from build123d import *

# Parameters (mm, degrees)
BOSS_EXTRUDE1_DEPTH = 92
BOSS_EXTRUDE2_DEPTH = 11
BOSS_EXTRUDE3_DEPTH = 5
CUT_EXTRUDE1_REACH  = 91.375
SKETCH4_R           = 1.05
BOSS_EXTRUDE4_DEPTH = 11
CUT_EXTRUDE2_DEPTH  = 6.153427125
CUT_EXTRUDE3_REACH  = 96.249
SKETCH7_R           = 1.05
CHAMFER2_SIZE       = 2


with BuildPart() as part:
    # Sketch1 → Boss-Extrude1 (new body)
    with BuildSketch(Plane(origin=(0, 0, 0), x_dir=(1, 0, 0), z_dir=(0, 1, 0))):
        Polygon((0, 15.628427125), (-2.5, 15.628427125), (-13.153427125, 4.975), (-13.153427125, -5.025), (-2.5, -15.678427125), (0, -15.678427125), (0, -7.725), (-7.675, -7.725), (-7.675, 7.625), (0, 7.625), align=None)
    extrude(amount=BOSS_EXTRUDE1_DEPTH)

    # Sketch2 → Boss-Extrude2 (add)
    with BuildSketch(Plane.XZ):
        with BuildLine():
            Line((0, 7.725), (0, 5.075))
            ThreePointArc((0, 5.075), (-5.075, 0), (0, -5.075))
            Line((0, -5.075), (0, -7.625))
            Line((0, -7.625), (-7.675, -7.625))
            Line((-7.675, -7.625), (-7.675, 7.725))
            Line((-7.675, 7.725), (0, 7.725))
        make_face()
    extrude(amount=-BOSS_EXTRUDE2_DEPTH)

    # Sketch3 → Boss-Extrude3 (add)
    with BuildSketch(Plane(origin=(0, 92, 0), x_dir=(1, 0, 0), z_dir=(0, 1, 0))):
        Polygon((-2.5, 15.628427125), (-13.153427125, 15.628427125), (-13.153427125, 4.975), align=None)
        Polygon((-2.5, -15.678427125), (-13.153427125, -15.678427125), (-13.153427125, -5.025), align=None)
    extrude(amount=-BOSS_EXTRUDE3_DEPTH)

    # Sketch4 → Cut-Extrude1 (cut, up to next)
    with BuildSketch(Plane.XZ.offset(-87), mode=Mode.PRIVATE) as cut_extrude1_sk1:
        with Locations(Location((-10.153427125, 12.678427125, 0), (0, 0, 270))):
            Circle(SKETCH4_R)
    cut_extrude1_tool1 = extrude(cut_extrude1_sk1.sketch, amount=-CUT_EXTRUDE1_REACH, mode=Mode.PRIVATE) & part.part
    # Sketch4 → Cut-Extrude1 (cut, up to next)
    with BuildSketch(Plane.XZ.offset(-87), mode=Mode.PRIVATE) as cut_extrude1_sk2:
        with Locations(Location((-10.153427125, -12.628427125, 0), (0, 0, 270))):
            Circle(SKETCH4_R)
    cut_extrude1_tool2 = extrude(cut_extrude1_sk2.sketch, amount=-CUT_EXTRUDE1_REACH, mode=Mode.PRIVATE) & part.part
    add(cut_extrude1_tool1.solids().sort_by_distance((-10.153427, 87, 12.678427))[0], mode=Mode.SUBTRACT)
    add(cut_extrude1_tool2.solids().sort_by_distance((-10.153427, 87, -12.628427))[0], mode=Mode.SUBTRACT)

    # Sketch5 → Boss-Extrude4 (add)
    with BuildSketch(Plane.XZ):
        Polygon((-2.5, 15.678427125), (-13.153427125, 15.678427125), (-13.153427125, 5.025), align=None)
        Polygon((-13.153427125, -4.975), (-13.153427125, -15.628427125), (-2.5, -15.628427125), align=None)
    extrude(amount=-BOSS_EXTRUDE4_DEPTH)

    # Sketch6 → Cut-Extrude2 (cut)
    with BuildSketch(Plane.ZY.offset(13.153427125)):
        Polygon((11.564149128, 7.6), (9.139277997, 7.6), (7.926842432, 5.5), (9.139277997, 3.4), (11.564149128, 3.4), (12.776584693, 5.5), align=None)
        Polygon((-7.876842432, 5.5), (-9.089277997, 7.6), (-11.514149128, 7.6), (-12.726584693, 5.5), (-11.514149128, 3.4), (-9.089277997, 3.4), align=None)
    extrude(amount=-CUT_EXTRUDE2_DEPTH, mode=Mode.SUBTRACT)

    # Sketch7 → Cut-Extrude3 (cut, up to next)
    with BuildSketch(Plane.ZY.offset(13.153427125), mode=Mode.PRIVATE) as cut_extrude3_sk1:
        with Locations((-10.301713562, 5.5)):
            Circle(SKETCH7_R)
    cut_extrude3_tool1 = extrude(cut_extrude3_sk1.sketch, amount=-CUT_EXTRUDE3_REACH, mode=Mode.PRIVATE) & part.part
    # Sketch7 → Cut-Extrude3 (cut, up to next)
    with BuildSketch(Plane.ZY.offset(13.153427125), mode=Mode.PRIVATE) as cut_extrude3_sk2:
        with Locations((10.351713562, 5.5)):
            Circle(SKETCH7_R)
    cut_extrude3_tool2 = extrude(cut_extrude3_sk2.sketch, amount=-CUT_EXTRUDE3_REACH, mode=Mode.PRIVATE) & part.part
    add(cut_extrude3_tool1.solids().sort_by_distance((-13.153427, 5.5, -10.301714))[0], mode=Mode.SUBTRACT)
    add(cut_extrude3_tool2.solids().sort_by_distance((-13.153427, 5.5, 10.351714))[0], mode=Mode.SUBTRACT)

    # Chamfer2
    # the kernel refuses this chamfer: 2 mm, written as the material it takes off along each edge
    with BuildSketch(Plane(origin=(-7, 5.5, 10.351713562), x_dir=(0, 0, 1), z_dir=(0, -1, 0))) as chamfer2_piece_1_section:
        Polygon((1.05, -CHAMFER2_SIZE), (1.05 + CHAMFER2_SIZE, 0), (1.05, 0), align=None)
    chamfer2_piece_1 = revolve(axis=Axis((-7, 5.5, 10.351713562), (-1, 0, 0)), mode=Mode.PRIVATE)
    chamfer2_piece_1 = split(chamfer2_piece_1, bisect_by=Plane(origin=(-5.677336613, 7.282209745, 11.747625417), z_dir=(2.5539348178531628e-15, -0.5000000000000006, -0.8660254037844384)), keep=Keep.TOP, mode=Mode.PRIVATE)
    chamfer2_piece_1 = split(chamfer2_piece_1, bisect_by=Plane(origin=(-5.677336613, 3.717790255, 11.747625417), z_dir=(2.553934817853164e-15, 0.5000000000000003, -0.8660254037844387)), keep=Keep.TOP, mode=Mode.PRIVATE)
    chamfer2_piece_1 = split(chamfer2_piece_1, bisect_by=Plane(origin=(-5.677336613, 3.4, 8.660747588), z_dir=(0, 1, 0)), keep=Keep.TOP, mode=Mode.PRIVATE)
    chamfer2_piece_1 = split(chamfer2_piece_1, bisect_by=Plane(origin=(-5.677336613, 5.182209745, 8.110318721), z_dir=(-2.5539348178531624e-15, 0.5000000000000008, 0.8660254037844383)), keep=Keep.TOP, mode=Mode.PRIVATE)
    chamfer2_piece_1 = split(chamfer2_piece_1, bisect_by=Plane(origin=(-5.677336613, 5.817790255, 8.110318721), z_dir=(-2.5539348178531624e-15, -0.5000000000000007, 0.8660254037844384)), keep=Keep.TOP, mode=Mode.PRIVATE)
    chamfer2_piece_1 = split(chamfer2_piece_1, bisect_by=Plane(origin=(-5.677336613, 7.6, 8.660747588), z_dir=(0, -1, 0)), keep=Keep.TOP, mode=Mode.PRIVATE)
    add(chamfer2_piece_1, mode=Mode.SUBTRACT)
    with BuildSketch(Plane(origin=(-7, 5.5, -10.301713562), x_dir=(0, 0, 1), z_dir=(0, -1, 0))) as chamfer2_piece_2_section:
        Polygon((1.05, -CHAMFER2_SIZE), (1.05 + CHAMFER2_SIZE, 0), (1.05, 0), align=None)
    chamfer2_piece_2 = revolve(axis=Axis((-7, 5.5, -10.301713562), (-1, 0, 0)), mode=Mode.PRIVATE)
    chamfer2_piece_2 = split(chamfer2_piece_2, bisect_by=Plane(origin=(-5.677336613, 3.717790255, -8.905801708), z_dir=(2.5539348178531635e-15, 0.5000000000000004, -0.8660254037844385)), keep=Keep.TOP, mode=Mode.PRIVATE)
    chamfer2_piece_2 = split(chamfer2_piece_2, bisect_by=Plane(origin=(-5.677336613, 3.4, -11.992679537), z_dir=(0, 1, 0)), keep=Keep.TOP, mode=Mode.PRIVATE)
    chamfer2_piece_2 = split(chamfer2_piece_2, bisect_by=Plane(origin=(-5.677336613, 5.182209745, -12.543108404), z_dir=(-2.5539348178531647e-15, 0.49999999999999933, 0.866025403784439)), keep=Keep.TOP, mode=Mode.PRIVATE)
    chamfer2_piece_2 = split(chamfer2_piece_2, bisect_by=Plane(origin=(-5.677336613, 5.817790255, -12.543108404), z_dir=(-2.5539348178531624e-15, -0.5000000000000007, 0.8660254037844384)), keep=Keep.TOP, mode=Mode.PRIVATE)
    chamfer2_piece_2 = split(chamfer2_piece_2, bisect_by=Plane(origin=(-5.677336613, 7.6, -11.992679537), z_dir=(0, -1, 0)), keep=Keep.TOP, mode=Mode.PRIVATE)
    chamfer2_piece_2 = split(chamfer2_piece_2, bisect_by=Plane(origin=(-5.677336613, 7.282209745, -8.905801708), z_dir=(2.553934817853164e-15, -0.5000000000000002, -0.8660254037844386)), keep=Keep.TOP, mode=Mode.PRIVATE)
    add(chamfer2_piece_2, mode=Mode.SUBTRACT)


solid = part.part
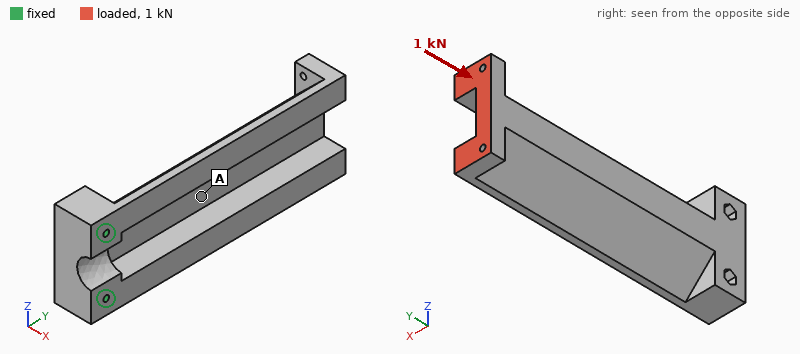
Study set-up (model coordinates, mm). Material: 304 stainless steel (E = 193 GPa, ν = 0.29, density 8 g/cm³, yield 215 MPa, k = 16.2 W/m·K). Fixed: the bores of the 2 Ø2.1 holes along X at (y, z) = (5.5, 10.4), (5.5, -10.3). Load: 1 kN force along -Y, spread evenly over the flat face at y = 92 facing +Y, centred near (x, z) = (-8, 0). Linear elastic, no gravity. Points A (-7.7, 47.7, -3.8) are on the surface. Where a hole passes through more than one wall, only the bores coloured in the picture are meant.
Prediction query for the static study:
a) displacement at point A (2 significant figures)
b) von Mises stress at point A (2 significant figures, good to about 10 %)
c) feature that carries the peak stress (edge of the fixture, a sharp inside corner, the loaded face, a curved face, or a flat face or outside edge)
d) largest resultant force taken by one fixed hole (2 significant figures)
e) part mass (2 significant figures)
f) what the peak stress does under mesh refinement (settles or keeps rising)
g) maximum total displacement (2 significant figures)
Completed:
14 µm
5.9 MPa
edge of the fixture
500 N
150 g
keeps rising
35 µm
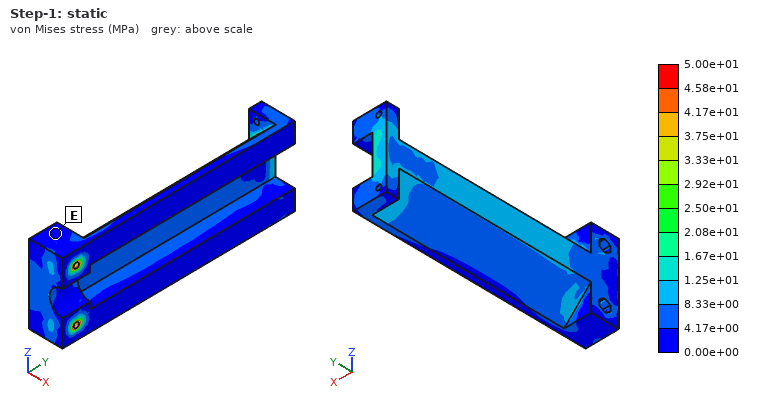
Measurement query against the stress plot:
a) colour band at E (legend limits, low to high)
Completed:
0.00e+00 to 4.17e+00 MPa
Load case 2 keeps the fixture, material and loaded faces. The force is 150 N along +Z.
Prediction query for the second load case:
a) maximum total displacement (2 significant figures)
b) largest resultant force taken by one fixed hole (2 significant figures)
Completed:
28 µm
600 N
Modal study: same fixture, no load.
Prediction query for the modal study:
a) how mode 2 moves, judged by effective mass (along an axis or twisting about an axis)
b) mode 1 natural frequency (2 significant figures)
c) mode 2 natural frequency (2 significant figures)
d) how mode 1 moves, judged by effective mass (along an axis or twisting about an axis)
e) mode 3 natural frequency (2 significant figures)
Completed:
along Z
870 Hz
1900 Hz
along X
3600 Hz
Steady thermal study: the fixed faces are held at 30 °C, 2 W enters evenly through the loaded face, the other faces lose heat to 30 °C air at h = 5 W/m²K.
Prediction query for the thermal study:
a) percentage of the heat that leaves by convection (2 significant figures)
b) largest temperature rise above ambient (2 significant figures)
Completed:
42 %
43 K
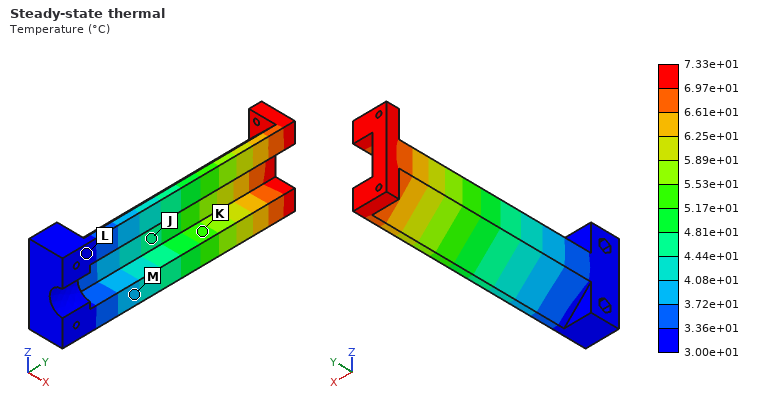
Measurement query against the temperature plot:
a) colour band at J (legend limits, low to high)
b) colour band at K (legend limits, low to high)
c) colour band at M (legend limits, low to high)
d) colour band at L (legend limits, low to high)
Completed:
4.44e+01 to 4.81e+01 °C
5.17e+01 to 5.53e+01 °C
3.72e+01 to 4.08e+01 °C
3.00e+01 to 3.36e+01 °C
